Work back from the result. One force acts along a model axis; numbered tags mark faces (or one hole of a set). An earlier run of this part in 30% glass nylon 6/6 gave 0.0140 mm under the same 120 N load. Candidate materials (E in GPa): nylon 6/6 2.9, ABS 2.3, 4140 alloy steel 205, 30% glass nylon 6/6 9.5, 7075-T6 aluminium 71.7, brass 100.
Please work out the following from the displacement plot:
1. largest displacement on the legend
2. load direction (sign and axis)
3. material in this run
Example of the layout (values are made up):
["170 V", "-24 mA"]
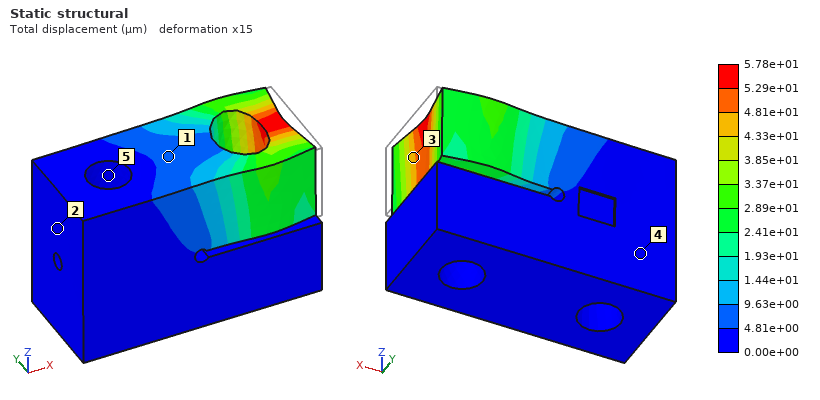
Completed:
["5.78e+01 µm", "-X", "ABS"]
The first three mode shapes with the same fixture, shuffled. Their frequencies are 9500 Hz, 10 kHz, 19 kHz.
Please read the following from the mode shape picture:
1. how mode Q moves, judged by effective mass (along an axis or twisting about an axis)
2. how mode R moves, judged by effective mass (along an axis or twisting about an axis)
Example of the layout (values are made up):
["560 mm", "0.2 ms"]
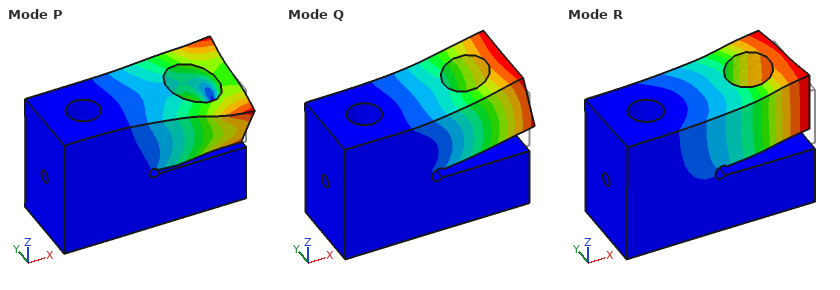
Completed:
["along Z", "along Y"]
